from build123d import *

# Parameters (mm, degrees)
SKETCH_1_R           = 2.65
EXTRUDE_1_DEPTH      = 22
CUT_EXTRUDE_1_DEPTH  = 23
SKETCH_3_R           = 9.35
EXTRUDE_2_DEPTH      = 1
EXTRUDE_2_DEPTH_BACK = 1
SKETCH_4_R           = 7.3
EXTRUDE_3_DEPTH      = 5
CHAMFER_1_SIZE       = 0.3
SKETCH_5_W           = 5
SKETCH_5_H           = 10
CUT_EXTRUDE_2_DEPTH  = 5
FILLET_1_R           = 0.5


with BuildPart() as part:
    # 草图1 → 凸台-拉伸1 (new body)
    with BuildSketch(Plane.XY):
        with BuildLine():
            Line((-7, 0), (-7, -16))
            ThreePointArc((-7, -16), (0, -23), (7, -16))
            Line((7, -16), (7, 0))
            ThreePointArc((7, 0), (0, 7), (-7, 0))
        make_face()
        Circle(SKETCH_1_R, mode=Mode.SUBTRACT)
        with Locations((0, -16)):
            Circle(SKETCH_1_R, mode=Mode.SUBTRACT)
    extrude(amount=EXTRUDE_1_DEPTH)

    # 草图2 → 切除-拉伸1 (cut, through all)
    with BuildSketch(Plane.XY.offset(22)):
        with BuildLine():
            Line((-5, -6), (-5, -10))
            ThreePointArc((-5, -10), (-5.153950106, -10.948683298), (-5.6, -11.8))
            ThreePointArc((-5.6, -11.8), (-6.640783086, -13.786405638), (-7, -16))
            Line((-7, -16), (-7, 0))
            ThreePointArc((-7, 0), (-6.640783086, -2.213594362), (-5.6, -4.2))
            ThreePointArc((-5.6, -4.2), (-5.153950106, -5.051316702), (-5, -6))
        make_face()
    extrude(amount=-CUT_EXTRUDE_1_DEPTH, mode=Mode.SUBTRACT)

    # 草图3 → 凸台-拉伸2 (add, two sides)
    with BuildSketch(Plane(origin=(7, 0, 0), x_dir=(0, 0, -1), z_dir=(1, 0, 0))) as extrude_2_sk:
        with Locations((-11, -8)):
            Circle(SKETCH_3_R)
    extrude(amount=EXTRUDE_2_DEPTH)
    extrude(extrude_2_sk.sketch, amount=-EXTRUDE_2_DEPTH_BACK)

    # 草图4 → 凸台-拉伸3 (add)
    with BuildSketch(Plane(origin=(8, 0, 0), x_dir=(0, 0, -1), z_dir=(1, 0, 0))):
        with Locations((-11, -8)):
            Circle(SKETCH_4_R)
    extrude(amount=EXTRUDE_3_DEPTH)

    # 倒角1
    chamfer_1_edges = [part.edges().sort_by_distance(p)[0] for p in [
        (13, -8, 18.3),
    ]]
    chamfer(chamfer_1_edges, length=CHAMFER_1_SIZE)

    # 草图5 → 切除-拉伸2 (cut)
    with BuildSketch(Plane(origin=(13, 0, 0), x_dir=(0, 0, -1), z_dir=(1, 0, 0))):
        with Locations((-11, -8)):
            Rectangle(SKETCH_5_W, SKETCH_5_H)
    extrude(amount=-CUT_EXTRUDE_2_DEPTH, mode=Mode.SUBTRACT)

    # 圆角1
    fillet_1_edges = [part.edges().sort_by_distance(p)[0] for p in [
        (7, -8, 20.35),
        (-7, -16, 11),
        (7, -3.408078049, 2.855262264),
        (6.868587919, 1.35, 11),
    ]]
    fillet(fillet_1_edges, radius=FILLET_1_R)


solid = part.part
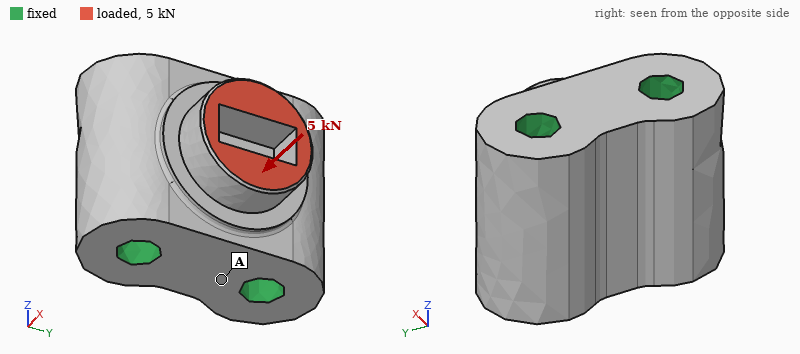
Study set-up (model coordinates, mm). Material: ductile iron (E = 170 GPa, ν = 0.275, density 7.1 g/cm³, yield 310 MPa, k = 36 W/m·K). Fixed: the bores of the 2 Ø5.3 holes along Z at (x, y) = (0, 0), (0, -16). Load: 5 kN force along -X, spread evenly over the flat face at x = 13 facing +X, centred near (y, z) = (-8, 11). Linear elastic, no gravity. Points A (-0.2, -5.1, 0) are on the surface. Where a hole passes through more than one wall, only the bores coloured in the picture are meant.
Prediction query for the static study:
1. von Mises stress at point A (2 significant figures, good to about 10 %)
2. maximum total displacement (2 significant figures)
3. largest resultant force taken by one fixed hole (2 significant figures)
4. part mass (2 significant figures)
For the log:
8.0 MPa
2.5 µm
2.7 kN
55 g
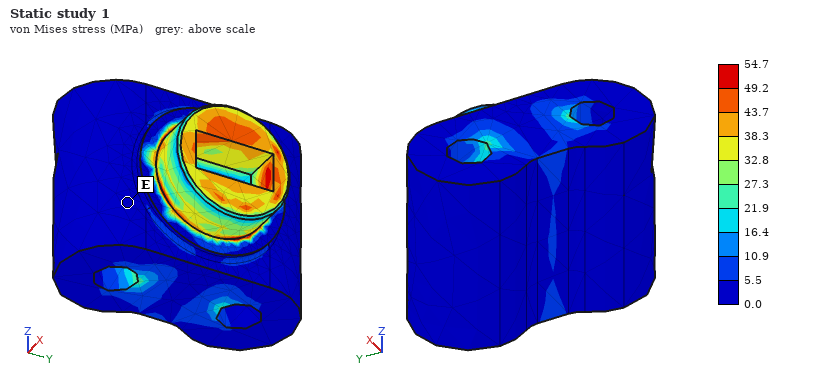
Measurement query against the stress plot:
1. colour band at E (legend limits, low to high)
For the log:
0.0 to 5.5 MPa
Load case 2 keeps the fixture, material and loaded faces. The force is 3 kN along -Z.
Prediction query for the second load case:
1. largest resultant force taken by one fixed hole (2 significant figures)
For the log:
1.5 kN
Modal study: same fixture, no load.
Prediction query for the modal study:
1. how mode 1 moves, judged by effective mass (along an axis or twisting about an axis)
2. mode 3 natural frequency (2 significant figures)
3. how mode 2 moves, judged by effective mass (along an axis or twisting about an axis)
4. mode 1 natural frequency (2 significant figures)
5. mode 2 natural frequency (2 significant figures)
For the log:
along Z
84 kHz
along Y
66 kHz
80 kHz
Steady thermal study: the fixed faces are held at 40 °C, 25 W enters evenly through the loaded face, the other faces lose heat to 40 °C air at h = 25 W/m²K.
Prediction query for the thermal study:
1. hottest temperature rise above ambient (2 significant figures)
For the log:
49 K
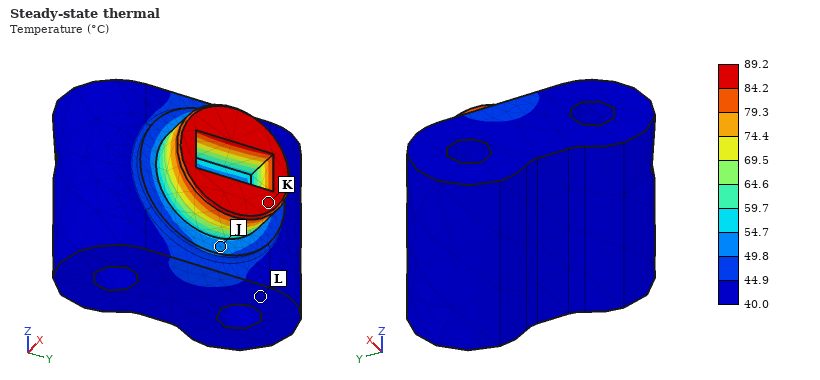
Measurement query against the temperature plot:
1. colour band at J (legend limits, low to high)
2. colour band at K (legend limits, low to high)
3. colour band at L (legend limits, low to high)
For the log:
49.8 to 54.7 °C
84.2 to 89.2 °C
40.0 to 44.9 °C
